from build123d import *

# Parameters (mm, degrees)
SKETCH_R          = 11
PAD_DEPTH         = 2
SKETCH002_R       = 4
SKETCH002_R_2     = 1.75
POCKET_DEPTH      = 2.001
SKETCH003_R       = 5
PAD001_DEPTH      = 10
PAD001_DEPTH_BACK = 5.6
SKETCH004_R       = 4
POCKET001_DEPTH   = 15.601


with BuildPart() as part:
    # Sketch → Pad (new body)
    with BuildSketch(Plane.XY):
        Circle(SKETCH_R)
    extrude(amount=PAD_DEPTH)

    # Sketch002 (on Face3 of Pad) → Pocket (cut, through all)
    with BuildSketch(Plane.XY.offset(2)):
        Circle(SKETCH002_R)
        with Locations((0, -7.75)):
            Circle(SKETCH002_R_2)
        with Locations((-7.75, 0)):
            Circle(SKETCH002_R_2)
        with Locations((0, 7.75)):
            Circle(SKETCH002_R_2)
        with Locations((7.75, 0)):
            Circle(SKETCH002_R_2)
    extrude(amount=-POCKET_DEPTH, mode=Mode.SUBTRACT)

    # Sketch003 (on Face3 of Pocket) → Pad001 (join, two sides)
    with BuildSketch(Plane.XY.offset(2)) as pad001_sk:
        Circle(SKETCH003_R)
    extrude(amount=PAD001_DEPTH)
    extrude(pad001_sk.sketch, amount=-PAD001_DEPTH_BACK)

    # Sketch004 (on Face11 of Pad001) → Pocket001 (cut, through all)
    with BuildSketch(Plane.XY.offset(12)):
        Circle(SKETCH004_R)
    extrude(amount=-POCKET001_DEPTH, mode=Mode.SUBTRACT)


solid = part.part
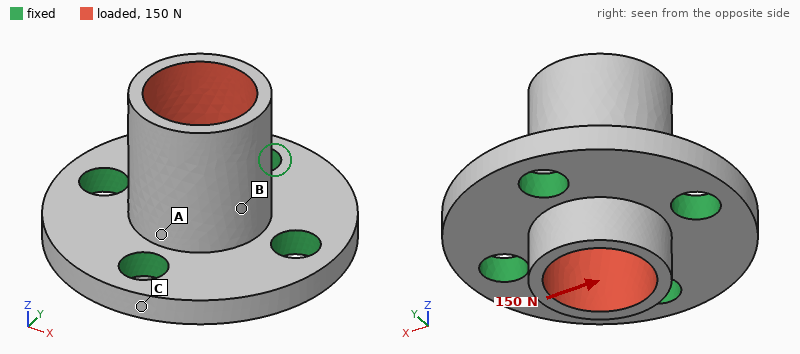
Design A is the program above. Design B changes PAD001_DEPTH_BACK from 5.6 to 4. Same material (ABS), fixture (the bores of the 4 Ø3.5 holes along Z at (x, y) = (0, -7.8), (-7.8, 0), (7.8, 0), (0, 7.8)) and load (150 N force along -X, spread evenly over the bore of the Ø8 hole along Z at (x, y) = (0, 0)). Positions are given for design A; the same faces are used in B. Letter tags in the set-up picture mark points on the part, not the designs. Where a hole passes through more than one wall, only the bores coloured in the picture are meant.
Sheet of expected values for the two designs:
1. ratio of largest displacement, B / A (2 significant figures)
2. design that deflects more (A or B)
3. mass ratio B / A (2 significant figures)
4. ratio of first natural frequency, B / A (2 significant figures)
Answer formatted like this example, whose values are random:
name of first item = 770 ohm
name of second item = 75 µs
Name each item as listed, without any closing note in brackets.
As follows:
ratio of largest displacement, B / A = 1.1
design that deflects more = B
mass ratio B / A = 0.95
ratio of first natural frequency, B / A = 1.00
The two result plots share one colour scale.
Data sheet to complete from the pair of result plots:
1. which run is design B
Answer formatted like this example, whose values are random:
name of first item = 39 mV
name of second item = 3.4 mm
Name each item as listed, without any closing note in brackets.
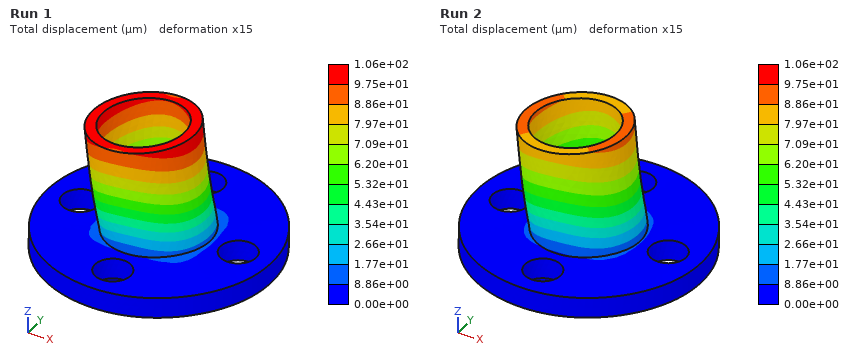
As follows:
which run is design B = Run 1
